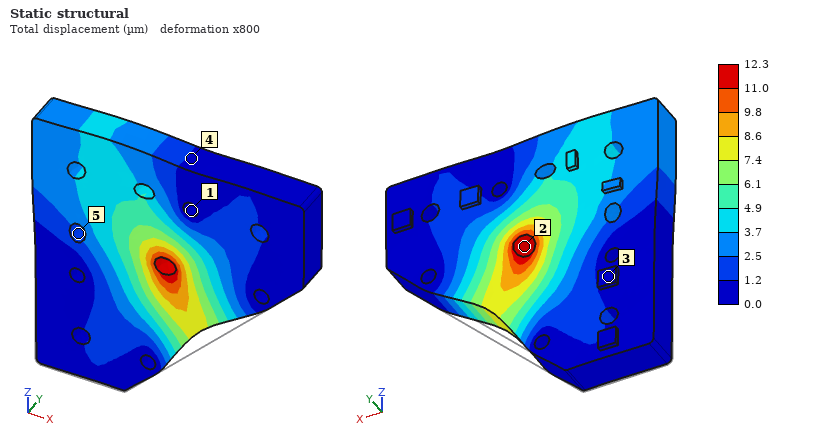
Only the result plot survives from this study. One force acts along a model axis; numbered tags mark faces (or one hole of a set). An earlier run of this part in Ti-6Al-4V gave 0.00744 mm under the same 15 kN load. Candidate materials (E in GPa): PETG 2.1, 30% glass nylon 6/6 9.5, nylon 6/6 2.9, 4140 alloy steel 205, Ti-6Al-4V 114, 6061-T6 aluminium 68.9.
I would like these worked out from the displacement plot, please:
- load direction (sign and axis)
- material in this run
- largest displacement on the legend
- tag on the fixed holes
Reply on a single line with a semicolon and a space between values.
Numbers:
+Z; 6061-T6 aluminium; 12.3 µm; 1
